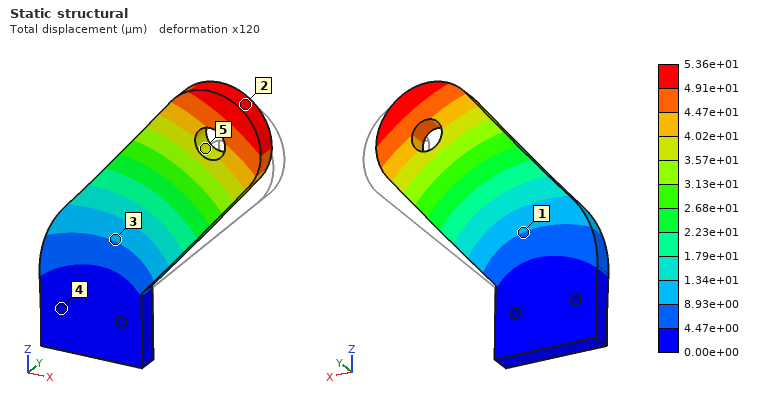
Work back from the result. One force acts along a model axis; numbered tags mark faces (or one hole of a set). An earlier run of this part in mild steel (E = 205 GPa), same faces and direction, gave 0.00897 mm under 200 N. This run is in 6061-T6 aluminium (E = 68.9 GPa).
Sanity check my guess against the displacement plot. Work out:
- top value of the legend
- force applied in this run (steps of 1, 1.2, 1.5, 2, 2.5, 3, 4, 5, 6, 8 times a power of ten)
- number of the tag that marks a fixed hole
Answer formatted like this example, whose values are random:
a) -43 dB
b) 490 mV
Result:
a) 5.36e+01 µm
b) 400 N
c) 4
